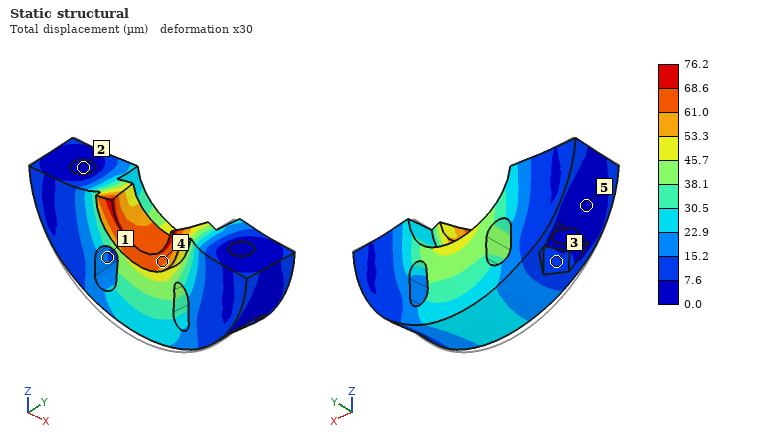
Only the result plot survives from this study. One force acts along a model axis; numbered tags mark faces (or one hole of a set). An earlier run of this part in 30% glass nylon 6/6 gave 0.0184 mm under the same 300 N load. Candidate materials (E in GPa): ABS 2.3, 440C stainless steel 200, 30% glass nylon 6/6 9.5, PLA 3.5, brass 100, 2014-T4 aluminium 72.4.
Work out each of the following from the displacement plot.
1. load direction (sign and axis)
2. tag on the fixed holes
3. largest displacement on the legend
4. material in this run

+Y
2
76.2 µm
ABS
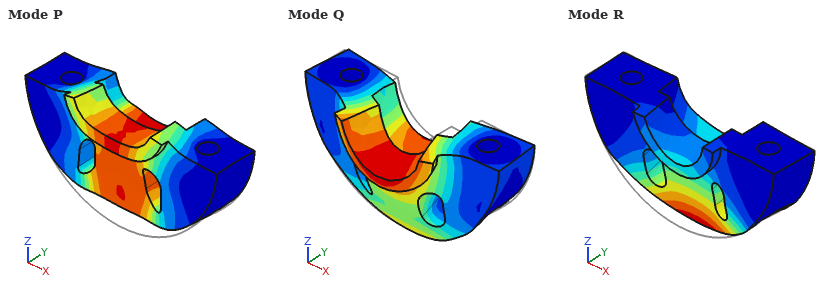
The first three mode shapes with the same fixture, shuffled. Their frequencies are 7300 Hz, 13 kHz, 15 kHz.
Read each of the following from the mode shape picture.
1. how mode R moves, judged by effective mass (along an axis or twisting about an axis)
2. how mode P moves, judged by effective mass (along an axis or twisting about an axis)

along Y
along Z
